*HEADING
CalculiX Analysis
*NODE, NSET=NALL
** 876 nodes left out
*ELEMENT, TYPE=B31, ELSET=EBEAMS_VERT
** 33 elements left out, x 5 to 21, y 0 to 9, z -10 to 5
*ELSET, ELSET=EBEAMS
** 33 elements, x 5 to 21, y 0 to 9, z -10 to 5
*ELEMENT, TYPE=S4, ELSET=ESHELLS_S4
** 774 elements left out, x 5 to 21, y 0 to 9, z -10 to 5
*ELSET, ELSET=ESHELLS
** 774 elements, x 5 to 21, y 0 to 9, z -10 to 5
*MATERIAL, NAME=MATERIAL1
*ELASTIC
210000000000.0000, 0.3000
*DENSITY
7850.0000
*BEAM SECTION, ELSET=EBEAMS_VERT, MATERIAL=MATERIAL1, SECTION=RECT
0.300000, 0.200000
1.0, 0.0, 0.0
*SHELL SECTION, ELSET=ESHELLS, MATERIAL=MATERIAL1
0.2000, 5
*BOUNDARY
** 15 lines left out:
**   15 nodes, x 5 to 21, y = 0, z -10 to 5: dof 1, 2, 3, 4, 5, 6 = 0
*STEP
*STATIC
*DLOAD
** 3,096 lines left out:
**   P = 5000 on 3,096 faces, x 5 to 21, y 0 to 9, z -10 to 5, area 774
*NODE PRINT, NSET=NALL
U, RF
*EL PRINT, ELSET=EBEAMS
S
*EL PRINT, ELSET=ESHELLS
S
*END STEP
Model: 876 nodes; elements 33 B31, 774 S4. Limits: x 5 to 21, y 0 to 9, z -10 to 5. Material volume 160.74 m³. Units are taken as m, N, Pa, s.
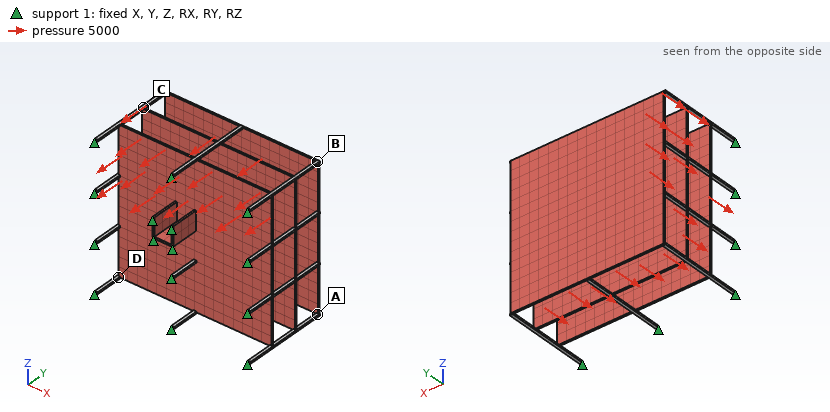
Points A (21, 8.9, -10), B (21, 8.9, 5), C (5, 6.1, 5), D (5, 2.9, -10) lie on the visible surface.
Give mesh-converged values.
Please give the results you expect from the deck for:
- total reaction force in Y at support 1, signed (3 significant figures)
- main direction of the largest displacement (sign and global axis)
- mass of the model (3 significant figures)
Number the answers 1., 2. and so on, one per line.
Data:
1. 1.44e+07 N
2. -Y
3. 1.26e+06 kg
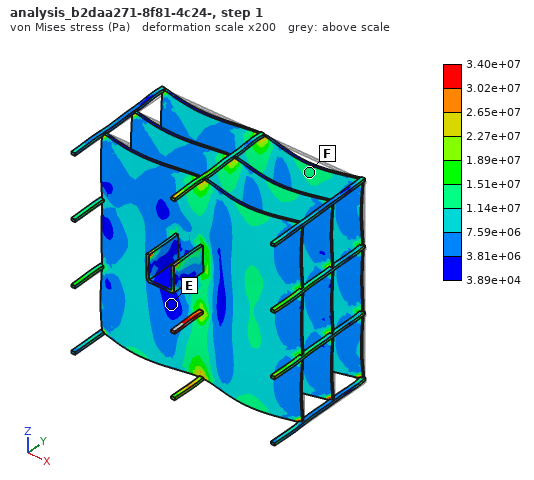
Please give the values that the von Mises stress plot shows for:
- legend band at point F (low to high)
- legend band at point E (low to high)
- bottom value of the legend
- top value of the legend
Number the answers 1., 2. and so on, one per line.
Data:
1. 1.14e+07 to 1.51e+07 Pa
2. 3.89e+04 to 3.81e+06 Pa
3. 3.89e+04 Pa
4. 3.40e+07 Pa
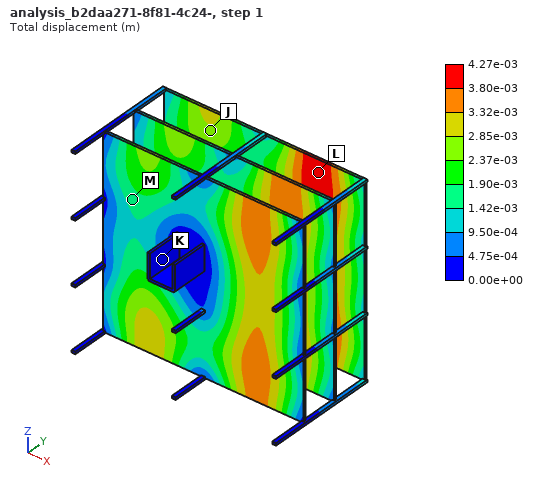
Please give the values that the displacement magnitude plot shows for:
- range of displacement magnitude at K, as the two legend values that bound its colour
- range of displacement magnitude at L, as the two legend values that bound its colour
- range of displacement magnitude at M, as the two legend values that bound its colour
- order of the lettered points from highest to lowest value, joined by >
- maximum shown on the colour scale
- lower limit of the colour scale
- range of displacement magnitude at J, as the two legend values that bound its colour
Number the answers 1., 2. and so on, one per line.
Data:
1. 0.00e+00 to 4.75e-04 m
2. 3.80e-03 to 4.27e-03 m
3. 1.42e-03 to 1.90e-03 m
4. L > J > M > K
5. 4.27e-03 m
6. 0.00e+00 m
7. 2.37e-03 to 2.85e-03 m
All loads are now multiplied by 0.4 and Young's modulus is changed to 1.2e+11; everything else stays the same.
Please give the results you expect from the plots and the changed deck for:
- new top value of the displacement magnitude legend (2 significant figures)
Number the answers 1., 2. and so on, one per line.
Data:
1. 0.0030 m
